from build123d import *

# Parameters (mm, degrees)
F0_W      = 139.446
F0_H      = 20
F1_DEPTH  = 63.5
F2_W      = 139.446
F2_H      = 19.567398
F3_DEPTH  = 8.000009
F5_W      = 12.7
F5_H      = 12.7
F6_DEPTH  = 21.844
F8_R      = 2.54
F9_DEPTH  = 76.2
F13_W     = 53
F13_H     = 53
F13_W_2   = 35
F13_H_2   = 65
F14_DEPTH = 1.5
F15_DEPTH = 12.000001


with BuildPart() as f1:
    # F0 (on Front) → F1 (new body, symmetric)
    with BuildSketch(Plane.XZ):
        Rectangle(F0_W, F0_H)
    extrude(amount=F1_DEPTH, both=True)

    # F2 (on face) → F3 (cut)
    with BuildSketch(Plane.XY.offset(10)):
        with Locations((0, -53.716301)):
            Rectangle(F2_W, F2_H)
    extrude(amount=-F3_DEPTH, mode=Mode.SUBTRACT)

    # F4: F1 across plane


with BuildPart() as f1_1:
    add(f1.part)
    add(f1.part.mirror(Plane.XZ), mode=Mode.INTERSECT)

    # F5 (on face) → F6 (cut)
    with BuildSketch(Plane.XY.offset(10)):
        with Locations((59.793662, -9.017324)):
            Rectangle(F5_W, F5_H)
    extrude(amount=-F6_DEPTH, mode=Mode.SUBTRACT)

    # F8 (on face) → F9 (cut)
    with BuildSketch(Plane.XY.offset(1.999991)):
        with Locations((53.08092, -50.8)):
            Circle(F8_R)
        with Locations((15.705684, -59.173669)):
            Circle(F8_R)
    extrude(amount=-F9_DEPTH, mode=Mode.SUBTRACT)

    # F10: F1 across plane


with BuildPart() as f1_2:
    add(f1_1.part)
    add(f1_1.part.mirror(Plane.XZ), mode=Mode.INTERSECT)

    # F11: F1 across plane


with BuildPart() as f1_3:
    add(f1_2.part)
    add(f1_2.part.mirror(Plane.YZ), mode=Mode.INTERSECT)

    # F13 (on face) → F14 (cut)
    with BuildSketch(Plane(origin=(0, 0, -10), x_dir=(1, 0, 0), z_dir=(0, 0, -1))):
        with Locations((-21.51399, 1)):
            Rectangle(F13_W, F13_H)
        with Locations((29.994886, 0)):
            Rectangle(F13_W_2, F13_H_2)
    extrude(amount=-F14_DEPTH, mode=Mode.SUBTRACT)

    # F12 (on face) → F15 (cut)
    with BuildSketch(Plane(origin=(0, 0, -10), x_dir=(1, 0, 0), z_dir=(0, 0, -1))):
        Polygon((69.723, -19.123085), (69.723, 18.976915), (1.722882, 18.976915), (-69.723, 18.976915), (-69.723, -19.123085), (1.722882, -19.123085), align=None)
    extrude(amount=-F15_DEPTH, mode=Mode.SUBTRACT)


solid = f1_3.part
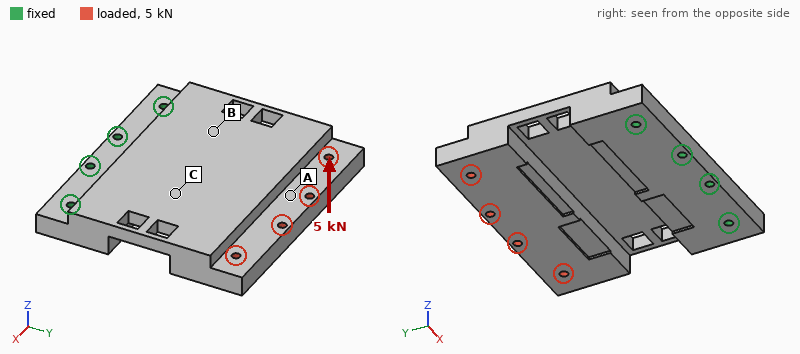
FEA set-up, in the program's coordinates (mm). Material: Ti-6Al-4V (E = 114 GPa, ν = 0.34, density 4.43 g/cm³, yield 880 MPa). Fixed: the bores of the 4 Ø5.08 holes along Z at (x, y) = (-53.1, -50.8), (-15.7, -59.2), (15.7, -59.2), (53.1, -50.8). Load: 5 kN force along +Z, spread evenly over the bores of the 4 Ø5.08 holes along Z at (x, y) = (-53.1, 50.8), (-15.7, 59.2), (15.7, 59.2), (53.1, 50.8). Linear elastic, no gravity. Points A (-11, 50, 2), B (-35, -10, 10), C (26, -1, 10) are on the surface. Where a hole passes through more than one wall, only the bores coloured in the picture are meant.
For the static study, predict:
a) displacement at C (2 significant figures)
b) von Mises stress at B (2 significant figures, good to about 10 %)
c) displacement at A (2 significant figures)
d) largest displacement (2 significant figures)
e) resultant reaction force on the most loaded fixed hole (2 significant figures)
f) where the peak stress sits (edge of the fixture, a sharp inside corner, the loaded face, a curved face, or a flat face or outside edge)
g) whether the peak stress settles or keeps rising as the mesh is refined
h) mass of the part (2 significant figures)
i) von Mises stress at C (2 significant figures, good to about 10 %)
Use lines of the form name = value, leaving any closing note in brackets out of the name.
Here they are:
displacement at C = 0.40 mm
von Mises stress at B = 230 MPa
displacement at A = 1.6 mm
largest displacement = 2.0 mm
resultant reaction force on the most loaded fixed hole = 2.9 kN
where the peak stress sits = edge of the fixture
whether the peak stress settles or keeps rising as the mesh is refined = keeps rising
mass of the part = 1.1 kg
von Mises stress at C = 200 MPa
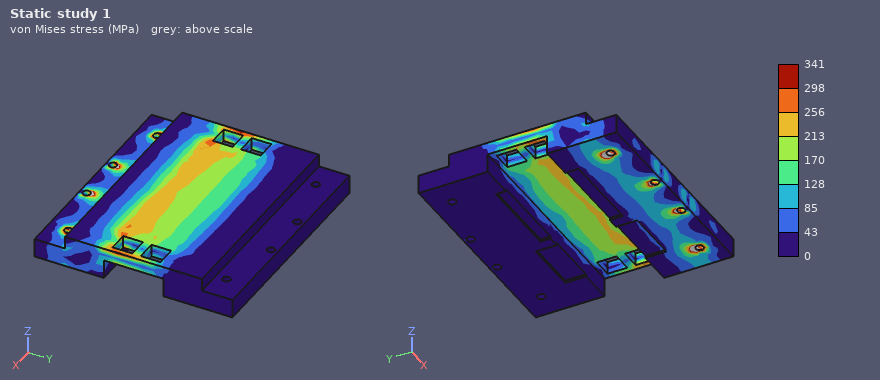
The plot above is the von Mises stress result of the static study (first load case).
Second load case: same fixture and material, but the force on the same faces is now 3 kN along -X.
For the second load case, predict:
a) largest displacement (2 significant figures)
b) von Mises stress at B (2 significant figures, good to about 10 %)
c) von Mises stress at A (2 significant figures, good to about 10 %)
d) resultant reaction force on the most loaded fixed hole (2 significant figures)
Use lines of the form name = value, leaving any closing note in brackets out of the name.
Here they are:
largest displacement = 56 µm
von Mises stress at B = 5.5 MPa
von Mises stress at A = 3.5 MPa
resultant reaction force on the most loaded fixed hole = 3.0 kN
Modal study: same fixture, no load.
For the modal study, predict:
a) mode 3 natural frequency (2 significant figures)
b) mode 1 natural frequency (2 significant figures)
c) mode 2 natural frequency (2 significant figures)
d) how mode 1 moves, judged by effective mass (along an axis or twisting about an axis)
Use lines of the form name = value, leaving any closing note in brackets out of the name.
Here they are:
mode 3 natural frequency = 2600 Hz
mode 1 natural frequency = 510 Hz
mode 2 natural frequency = 1300 Hz
how mode 1 moves, judged by effective mass = along Z
